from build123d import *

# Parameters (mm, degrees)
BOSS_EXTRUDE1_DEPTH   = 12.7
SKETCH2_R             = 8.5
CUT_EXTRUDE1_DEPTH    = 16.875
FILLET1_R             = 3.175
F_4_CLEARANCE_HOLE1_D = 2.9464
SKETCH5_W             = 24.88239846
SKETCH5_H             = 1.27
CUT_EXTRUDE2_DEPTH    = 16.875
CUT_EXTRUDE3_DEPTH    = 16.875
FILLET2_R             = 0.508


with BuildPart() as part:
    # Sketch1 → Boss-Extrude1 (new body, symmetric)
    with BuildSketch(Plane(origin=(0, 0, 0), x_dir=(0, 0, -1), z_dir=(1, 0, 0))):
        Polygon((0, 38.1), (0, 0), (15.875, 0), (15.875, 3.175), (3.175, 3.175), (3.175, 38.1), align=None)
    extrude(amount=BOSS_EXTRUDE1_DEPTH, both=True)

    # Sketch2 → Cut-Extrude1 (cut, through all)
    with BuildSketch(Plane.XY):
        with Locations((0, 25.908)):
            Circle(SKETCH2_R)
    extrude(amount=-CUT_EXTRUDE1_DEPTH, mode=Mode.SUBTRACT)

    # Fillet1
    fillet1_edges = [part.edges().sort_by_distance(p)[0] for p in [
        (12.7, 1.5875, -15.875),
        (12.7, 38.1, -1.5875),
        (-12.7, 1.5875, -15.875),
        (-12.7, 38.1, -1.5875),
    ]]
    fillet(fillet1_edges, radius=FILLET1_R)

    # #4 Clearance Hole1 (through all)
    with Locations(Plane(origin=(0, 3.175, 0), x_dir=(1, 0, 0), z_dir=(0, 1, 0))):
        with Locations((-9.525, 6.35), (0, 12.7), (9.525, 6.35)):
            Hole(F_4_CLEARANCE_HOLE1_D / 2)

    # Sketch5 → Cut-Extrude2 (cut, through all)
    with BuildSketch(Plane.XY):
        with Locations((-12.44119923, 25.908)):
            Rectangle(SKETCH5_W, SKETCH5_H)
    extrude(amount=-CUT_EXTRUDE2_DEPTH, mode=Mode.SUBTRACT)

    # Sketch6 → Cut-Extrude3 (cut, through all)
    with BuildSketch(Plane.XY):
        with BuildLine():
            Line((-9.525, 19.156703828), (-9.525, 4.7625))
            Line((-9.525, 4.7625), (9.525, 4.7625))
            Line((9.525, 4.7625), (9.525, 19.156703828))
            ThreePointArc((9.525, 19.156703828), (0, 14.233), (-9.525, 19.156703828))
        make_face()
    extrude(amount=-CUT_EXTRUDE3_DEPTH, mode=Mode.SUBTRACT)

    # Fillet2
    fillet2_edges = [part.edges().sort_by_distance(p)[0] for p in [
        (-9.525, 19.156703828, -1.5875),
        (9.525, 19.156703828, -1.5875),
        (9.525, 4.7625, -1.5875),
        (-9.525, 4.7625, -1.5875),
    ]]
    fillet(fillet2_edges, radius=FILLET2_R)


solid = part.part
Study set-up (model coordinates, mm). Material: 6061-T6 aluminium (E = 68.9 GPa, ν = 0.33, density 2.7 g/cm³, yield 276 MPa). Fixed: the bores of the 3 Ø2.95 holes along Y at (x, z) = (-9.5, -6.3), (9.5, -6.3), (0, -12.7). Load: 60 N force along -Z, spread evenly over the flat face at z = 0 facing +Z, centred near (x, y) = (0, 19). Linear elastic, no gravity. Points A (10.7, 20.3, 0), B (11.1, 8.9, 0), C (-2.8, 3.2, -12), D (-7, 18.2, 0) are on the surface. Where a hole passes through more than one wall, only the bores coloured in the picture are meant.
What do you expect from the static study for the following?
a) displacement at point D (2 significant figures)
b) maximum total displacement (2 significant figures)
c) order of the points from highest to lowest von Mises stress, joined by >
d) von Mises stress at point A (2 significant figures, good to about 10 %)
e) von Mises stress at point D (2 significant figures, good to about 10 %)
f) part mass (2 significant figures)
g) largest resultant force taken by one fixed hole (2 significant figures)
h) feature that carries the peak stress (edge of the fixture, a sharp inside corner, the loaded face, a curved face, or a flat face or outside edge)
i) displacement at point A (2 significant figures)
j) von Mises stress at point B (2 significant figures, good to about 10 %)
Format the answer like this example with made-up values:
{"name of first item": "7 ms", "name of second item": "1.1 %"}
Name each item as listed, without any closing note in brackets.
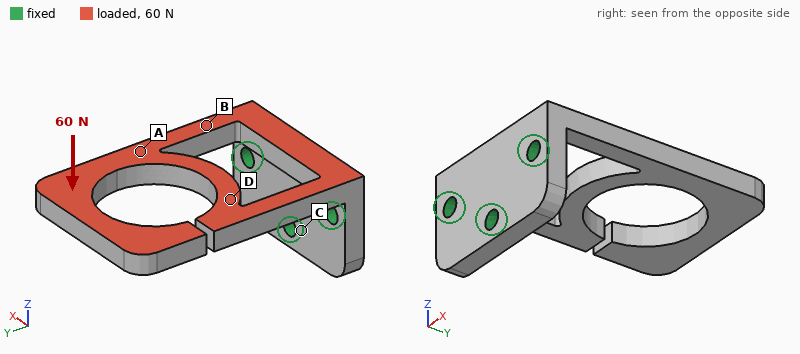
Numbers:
{"displacement at point D": "0.095 mm", "maximum total displacement": "0.54 mm", "order of the points from highest to lowest von Mises stress, joined by >": "B > A > D > C", "von Mises stress at point A": "44 MPa", "von Mises stress at point D": "16 MPa", "part mass": "7.0 g", "largest resultant force taken by one fixed hole": "29 N", "feature that carries the peak stress": "the loaded face", "displacement at point A": "0.15 mm", "von Mises stress at point B": "82 MPa"}
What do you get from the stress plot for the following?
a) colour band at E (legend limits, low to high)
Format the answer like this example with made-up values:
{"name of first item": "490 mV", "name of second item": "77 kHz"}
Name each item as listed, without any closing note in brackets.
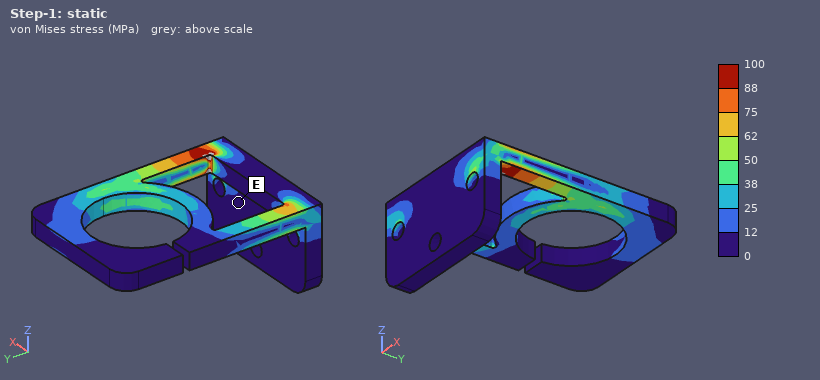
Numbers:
{"colour band at E": "0 to 12 MPa"}
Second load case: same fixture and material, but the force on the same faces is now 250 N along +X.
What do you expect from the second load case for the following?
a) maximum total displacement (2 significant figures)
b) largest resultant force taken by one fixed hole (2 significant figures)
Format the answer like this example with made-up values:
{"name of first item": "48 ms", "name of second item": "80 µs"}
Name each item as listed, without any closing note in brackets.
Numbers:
{"maximum total displacement": "0.50 mm", "largest resultant force taken by one fixed hole": "230 N"}
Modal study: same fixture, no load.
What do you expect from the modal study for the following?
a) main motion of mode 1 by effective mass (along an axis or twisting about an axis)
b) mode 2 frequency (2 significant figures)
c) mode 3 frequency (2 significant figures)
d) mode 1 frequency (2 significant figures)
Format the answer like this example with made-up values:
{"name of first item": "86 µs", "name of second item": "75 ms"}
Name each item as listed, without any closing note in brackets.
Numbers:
{"main motion of mode 1 by effective mass": "along Z", "mode 2 frequency": "1800 Hz", "mode 3 frequency": "2500 Hz", "mode 1 frequency": "970 Hz"}
